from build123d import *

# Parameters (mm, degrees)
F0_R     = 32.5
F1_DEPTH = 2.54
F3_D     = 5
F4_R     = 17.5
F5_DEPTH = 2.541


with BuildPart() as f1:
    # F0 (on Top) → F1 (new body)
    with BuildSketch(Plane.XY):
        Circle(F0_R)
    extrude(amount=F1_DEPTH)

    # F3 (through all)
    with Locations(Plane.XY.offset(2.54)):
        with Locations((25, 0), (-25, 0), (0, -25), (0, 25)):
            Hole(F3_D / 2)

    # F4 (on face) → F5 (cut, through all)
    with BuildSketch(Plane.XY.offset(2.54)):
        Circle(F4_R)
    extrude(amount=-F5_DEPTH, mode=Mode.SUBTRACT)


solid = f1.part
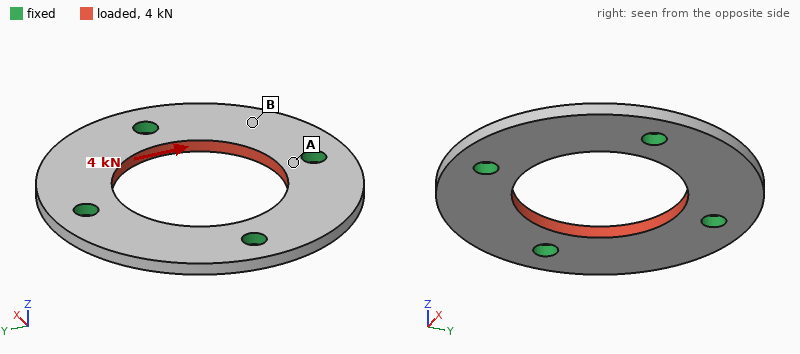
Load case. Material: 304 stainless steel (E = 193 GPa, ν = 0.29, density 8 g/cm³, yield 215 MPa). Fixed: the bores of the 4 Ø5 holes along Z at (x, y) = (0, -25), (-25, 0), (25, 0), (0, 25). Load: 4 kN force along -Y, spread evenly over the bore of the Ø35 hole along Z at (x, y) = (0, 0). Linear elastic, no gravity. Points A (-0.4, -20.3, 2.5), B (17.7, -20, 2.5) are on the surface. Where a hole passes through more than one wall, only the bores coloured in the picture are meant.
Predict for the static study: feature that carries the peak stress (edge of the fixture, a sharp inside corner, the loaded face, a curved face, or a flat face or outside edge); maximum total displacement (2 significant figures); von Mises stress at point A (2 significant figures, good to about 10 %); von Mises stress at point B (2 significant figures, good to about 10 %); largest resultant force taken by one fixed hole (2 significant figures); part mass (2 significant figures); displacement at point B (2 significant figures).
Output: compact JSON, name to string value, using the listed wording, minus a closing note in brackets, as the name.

{"feature that carries the peak stress": "edge of the fixture", "maximum total displacement": "2.5 µm", "von Mises stress at point A": "30 MPa", "von Mises stress at point B": "9.9 MPa", "largest resultant force taken by one fixed hole": "1.1 kN", "part mass": "46 g", "displacement at point B": "1.9 µm"}
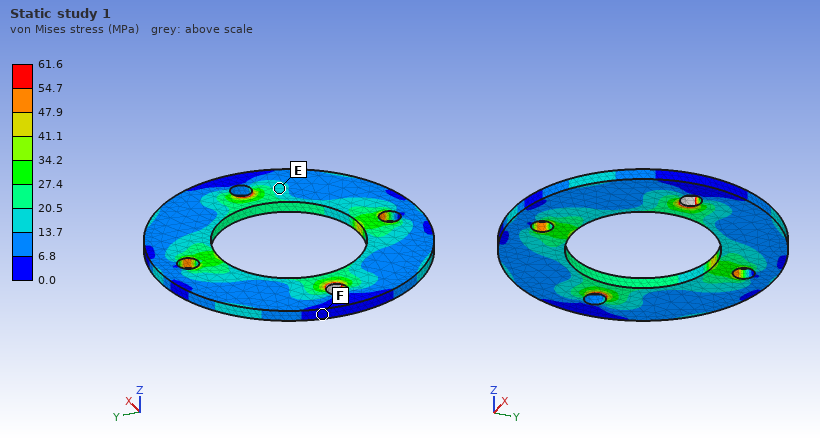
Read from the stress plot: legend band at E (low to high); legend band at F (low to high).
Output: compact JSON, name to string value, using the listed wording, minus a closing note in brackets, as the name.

{"legend band at E": "13.7 to 20.5 MPa", "legend band at F": "0.0 to 6.8 MPa"}
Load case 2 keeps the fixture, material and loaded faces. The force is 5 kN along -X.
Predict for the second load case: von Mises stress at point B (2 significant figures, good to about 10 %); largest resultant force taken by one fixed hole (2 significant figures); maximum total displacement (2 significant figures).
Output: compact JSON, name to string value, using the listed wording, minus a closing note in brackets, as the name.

{"von Mises stress at point B": "13 MPa", "largest resultant force taken by one fixed hole": "1.4 kN", "maximum total displacement": "3.1 µm"}
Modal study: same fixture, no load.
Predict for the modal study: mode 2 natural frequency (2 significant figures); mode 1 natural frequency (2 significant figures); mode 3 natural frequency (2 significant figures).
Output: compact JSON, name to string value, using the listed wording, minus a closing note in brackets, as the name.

{"mode 2 natural frequency": "7800 Hz", "mode 1 natural frequency": "7700 Hz", "mode 3 natural frequency": "7800 Hz"}
